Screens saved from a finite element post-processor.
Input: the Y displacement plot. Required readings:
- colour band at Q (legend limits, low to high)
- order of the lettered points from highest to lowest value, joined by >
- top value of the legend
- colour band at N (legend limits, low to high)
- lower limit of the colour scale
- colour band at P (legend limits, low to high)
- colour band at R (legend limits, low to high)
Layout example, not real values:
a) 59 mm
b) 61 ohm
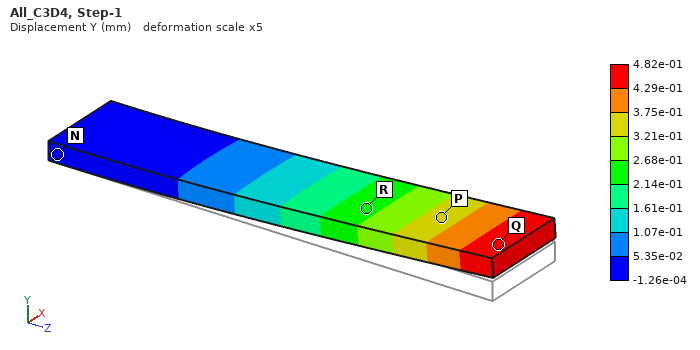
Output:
a) 4.29e-01 to 4.82e-01 mm
b) Q > P > R > N
c) 4.82e-01 mm
d) -1.26e-04 to 5.35e-02 mm
e) -1.26e-04 mm
f) 3.21e-01 to 3.75e-01 mm
g) 2.14e-01 to 2.68e-01 mm
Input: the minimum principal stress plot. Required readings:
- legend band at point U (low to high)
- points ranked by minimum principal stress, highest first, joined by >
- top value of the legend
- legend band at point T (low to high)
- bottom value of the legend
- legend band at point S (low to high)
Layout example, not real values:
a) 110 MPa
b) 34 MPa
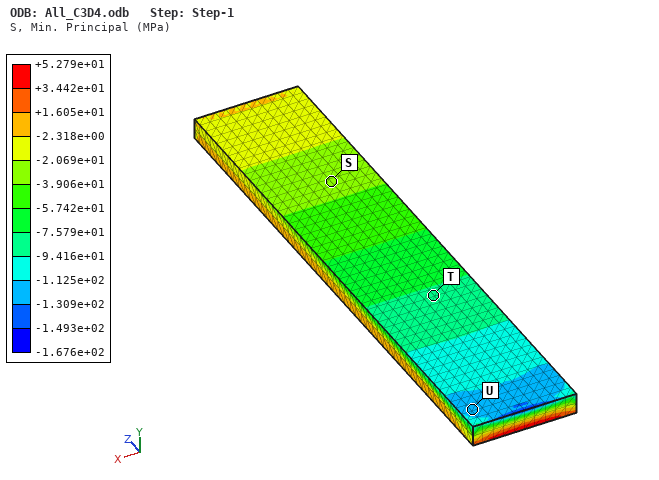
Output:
a) -1.309e+02 to -1.125e+02 MPa
b) S > T > U
c) +5.279e+01 MPa
d) -9.416e+01 to -7.579e+01 MPa
e) -1.676e+02 MPa
f) -3.906e+01 to -2.069e+01 MPa
